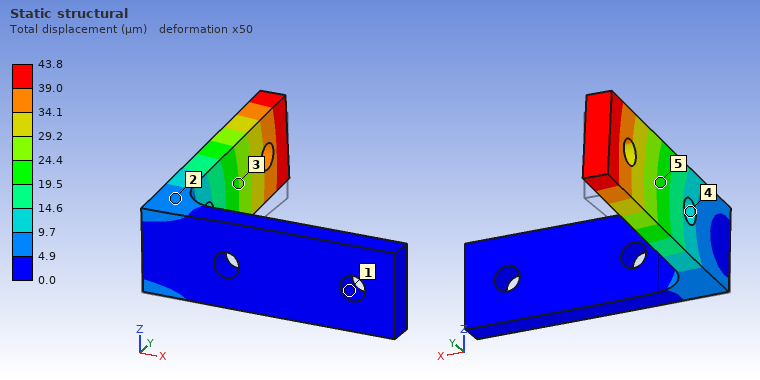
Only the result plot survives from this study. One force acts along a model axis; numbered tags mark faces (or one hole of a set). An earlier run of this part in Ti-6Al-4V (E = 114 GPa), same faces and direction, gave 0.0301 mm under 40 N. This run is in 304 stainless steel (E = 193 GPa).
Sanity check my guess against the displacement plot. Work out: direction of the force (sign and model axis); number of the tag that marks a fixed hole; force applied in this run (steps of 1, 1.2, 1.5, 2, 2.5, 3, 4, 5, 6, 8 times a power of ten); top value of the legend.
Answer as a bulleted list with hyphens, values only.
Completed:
- +Z
- 1
- 100 N
- 43.8 µm
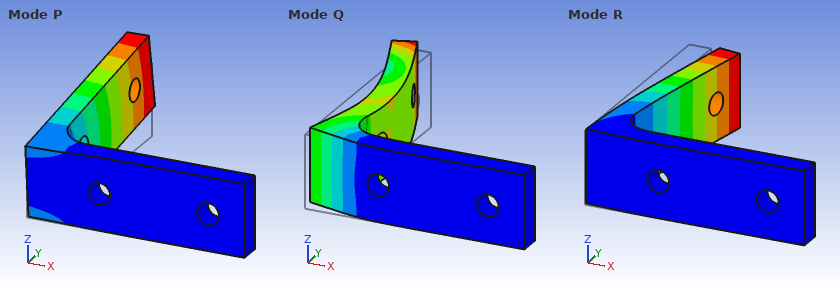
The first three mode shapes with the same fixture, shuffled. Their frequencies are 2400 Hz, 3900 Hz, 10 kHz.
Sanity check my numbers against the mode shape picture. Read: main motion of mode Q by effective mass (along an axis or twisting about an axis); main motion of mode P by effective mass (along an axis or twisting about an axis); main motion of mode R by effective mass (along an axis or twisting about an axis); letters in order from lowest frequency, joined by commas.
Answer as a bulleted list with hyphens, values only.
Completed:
- along Y
- along Z
- along X
- R, P, Q
